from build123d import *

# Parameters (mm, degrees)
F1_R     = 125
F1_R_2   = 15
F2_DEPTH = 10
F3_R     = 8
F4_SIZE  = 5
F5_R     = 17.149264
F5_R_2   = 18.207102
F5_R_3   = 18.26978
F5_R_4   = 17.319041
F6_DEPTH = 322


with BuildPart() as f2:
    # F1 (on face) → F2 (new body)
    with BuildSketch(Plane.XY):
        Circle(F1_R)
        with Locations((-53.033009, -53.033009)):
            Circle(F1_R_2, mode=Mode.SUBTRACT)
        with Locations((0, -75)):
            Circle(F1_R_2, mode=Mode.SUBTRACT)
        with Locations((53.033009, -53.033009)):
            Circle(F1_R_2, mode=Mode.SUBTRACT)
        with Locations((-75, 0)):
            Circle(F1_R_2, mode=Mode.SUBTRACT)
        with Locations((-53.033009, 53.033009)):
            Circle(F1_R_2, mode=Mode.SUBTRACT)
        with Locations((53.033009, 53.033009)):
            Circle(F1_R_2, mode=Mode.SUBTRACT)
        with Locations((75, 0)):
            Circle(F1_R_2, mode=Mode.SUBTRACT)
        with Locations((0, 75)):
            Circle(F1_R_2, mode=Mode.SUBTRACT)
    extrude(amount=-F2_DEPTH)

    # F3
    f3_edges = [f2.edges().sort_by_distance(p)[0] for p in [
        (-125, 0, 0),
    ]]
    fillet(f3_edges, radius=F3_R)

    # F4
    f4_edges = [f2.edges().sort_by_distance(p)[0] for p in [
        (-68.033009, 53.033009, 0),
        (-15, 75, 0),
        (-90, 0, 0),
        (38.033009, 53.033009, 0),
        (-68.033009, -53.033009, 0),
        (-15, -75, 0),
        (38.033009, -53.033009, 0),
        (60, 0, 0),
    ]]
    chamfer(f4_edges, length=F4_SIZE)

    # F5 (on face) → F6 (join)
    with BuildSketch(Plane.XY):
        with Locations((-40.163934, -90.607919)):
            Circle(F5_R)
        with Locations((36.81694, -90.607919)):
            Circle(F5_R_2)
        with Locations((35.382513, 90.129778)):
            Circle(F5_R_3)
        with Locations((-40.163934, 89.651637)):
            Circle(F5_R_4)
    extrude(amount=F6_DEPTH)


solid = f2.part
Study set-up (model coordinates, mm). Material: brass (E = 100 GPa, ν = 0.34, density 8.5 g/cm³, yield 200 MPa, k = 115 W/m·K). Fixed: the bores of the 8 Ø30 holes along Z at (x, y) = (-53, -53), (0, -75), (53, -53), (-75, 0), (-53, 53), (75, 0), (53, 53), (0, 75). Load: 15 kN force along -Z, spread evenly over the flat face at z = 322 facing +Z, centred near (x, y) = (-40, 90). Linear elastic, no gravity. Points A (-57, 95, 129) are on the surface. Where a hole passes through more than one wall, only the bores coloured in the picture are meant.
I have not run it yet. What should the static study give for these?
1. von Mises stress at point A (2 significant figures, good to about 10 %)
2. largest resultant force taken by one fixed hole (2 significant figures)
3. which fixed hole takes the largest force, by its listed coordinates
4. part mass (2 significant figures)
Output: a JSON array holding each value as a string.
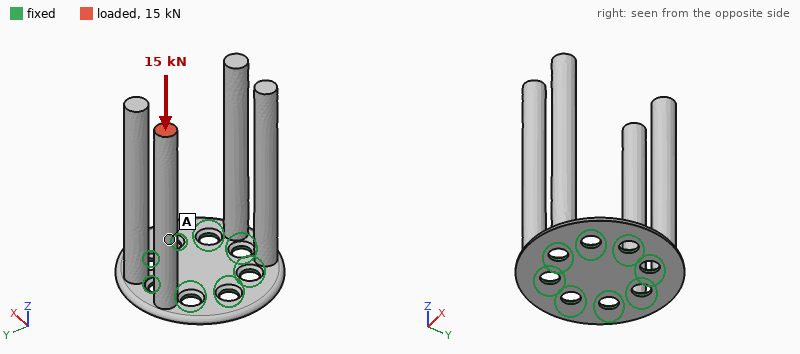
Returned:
["16 MPa", "9.2 kN", "(-53, 53)", "14 kg"]
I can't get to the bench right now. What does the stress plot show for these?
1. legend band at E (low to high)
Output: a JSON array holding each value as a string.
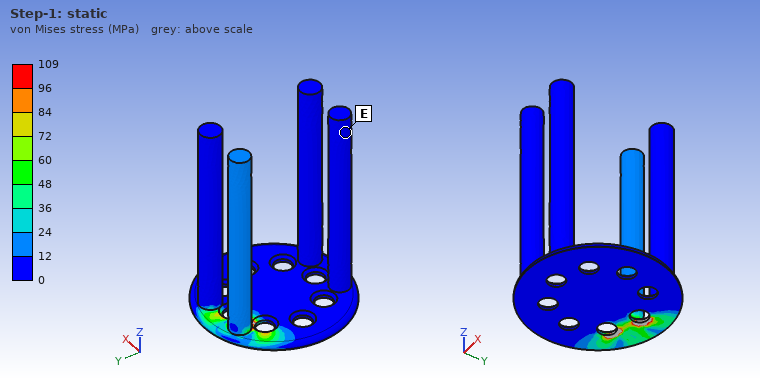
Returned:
["0 to 12 MPa"]
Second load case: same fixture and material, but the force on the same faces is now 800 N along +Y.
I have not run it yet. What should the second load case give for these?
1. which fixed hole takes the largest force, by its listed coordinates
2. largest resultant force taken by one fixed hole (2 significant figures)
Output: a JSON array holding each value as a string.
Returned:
["(0, 75)", "3.6 kN"]
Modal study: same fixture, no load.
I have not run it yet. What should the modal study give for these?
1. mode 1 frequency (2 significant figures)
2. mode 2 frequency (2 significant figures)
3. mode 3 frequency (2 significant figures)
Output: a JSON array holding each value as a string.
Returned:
["95 Hz", "97 Hz", "99 Hz"]
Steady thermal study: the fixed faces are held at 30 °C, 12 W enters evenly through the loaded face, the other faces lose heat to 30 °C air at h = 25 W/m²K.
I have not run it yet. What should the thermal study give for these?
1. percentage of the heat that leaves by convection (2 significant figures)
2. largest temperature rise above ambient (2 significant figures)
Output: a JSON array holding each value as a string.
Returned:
["67 %", "21 K"]
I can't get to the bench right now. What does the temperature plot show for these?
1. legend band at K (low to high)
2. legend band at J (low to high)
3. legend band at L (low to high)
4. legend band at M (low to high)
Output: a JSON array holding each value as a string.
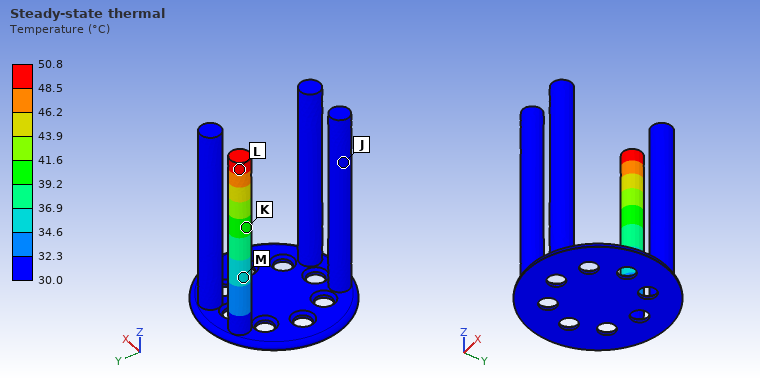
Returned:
["39.2 to 41.6 °C", "30.0 to 32.3 °C", "48.5 to 50.8 °C", "34.6 to 36.9 °C"]
